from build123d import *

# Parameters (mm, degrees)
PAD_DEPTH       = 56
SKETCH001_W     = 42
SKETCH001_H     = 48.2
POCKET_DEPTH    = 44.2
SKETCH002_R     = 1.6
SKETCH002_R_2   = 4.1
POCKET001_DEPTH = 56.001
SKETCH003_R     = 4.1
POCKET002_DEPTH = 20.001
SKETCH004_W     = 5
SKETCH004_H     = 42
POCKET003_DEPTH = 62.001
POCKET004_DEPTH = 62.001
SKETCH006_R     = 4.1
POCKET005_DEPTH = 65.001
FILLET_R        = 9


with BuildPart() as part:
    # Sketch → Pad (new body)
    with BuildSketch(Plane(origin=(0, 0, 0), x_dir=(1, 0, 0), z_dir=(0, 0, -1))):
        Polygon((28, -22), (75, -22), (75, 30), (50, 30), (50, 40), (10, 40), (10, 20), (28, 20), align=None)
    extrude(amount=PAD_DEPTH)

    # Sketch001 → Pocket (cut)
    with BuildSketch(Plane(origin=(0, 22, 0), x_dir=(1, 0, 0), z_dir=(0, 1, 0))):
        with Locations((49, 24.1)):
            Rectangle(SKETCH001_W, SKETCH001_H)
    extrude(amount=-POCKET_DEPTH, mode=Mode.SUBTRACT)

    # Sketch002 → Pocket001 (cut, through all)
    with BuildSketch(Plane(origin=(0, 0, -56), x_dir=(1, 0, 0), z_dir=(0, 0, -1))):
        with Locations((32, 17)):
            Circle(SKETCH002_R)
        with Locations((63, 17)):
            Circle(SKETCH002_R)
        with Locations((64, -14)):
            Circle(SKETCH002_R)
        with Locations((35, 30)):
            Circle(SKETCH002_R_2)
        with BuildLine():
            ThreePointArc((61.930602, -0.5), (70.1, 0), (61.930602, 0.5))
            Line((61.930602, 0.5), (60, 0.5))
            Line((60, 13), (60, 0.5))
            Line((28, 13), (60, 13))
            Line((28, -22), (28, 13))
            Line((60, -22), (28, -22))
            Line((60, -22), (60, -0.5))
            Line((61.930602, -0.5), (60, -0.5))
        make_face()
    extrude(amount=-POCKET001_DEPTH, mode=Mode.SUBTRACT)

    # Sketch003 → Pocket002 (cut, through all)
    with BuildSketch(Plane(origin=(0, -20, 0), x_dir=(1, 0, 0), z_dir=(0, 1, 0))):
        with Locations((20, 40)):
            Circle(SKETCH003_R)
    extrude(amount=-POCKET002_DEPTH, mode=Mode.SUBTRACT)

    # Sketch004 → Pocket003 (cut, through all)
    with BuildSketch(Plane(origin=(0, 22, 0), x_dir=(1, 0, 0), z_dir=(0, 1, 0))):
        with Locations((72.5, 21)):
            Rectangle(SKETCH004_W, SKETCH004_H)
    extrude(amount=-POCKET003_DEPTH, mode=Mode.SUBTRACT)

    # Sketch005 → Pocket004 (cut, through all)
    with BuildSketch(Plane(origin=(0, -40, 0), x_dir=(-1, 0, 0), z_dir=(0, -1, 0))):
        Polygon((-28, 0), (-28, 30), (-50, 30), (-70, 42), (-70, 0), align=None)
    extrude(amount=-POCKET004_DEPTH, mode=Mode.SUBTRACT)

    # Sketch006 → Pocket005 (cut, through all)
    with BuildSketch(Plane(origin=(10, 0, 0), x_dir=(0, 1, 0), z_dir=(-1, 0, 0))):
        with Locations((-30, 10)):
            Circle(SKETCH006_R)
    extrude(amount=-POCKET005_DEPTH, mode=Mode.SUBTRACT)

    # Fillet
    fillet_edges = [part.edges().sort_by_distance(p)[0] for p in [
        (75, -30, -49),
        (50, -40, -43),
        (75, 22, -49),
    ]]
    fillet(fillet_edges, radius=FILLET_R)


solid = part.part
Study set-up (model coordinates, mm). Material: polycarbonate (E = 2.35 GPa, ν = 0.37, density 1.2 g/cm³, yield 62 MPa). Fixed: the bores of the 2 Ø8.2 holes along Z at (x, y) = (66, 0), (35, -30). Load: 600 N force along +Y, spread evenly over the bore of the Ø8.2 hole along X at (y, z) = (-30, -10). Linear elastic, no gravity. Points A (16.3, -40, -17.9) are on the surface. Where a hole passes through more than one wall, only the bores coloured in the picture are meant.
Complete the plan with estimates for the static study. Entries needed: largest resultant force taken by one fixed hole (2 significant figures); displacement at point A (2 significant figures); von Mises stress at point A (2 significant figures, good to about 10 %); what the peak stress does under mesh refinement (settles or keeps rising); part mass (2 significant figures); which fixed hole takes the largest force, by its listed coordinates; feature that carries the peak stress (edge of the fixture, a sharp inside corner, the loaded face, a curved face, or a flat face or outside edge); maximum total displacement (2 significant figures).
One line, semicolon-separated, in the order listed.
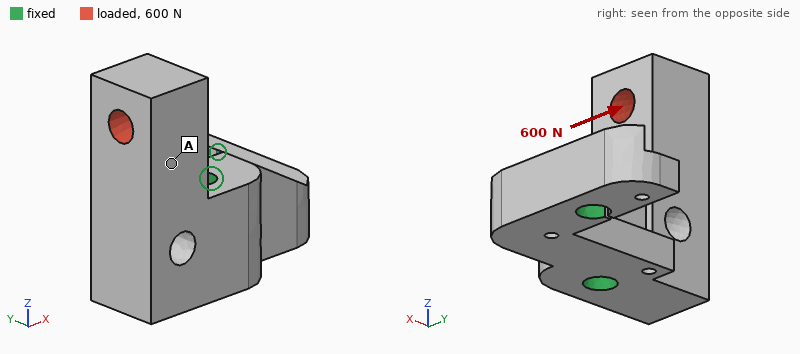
630 N; 0.42 mm; 4.7 MPa; keeps rising; 46 g; (35, -30); edge of the fixture; 0.78 mm
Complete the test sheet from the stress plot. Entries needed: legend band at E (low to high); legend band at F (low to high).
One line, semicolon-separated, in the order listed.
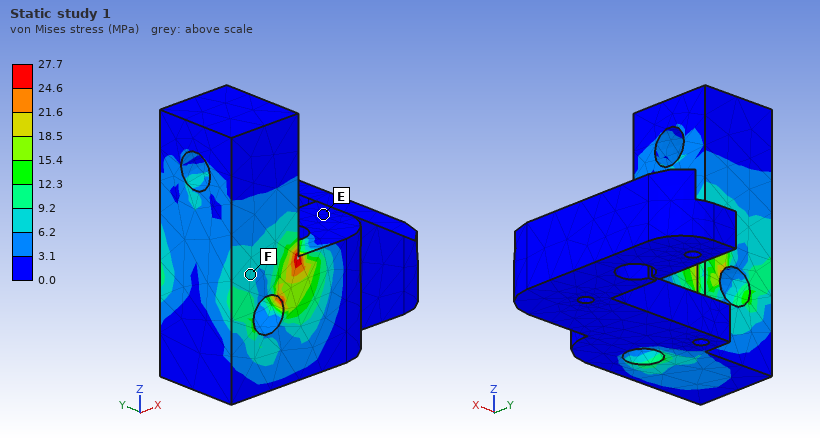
0.0 to 3.1 MPa; 6.2 to 9.2 MPa
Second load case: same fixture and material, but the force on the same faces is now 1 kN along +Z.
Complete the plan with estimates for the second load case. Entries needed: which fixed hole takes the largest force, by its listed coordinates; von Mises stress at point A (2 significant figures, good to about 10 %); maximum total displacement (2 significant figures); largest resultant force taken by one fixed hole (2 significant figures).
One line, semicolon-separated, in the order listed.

(35, -30); 2.6 MPa; 0.23 mm; 1.0 kN
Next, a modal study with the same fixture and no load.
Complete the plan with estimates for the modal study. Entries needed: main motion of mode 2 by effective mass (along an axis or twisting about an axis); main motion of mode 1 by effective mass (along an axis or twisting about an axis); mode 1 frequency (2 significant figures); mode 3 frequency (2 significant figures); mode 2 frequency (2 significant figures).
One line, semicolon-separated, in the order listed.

along X; along Y; 1700 Hz; 3600 Hz; 2000 Hz
